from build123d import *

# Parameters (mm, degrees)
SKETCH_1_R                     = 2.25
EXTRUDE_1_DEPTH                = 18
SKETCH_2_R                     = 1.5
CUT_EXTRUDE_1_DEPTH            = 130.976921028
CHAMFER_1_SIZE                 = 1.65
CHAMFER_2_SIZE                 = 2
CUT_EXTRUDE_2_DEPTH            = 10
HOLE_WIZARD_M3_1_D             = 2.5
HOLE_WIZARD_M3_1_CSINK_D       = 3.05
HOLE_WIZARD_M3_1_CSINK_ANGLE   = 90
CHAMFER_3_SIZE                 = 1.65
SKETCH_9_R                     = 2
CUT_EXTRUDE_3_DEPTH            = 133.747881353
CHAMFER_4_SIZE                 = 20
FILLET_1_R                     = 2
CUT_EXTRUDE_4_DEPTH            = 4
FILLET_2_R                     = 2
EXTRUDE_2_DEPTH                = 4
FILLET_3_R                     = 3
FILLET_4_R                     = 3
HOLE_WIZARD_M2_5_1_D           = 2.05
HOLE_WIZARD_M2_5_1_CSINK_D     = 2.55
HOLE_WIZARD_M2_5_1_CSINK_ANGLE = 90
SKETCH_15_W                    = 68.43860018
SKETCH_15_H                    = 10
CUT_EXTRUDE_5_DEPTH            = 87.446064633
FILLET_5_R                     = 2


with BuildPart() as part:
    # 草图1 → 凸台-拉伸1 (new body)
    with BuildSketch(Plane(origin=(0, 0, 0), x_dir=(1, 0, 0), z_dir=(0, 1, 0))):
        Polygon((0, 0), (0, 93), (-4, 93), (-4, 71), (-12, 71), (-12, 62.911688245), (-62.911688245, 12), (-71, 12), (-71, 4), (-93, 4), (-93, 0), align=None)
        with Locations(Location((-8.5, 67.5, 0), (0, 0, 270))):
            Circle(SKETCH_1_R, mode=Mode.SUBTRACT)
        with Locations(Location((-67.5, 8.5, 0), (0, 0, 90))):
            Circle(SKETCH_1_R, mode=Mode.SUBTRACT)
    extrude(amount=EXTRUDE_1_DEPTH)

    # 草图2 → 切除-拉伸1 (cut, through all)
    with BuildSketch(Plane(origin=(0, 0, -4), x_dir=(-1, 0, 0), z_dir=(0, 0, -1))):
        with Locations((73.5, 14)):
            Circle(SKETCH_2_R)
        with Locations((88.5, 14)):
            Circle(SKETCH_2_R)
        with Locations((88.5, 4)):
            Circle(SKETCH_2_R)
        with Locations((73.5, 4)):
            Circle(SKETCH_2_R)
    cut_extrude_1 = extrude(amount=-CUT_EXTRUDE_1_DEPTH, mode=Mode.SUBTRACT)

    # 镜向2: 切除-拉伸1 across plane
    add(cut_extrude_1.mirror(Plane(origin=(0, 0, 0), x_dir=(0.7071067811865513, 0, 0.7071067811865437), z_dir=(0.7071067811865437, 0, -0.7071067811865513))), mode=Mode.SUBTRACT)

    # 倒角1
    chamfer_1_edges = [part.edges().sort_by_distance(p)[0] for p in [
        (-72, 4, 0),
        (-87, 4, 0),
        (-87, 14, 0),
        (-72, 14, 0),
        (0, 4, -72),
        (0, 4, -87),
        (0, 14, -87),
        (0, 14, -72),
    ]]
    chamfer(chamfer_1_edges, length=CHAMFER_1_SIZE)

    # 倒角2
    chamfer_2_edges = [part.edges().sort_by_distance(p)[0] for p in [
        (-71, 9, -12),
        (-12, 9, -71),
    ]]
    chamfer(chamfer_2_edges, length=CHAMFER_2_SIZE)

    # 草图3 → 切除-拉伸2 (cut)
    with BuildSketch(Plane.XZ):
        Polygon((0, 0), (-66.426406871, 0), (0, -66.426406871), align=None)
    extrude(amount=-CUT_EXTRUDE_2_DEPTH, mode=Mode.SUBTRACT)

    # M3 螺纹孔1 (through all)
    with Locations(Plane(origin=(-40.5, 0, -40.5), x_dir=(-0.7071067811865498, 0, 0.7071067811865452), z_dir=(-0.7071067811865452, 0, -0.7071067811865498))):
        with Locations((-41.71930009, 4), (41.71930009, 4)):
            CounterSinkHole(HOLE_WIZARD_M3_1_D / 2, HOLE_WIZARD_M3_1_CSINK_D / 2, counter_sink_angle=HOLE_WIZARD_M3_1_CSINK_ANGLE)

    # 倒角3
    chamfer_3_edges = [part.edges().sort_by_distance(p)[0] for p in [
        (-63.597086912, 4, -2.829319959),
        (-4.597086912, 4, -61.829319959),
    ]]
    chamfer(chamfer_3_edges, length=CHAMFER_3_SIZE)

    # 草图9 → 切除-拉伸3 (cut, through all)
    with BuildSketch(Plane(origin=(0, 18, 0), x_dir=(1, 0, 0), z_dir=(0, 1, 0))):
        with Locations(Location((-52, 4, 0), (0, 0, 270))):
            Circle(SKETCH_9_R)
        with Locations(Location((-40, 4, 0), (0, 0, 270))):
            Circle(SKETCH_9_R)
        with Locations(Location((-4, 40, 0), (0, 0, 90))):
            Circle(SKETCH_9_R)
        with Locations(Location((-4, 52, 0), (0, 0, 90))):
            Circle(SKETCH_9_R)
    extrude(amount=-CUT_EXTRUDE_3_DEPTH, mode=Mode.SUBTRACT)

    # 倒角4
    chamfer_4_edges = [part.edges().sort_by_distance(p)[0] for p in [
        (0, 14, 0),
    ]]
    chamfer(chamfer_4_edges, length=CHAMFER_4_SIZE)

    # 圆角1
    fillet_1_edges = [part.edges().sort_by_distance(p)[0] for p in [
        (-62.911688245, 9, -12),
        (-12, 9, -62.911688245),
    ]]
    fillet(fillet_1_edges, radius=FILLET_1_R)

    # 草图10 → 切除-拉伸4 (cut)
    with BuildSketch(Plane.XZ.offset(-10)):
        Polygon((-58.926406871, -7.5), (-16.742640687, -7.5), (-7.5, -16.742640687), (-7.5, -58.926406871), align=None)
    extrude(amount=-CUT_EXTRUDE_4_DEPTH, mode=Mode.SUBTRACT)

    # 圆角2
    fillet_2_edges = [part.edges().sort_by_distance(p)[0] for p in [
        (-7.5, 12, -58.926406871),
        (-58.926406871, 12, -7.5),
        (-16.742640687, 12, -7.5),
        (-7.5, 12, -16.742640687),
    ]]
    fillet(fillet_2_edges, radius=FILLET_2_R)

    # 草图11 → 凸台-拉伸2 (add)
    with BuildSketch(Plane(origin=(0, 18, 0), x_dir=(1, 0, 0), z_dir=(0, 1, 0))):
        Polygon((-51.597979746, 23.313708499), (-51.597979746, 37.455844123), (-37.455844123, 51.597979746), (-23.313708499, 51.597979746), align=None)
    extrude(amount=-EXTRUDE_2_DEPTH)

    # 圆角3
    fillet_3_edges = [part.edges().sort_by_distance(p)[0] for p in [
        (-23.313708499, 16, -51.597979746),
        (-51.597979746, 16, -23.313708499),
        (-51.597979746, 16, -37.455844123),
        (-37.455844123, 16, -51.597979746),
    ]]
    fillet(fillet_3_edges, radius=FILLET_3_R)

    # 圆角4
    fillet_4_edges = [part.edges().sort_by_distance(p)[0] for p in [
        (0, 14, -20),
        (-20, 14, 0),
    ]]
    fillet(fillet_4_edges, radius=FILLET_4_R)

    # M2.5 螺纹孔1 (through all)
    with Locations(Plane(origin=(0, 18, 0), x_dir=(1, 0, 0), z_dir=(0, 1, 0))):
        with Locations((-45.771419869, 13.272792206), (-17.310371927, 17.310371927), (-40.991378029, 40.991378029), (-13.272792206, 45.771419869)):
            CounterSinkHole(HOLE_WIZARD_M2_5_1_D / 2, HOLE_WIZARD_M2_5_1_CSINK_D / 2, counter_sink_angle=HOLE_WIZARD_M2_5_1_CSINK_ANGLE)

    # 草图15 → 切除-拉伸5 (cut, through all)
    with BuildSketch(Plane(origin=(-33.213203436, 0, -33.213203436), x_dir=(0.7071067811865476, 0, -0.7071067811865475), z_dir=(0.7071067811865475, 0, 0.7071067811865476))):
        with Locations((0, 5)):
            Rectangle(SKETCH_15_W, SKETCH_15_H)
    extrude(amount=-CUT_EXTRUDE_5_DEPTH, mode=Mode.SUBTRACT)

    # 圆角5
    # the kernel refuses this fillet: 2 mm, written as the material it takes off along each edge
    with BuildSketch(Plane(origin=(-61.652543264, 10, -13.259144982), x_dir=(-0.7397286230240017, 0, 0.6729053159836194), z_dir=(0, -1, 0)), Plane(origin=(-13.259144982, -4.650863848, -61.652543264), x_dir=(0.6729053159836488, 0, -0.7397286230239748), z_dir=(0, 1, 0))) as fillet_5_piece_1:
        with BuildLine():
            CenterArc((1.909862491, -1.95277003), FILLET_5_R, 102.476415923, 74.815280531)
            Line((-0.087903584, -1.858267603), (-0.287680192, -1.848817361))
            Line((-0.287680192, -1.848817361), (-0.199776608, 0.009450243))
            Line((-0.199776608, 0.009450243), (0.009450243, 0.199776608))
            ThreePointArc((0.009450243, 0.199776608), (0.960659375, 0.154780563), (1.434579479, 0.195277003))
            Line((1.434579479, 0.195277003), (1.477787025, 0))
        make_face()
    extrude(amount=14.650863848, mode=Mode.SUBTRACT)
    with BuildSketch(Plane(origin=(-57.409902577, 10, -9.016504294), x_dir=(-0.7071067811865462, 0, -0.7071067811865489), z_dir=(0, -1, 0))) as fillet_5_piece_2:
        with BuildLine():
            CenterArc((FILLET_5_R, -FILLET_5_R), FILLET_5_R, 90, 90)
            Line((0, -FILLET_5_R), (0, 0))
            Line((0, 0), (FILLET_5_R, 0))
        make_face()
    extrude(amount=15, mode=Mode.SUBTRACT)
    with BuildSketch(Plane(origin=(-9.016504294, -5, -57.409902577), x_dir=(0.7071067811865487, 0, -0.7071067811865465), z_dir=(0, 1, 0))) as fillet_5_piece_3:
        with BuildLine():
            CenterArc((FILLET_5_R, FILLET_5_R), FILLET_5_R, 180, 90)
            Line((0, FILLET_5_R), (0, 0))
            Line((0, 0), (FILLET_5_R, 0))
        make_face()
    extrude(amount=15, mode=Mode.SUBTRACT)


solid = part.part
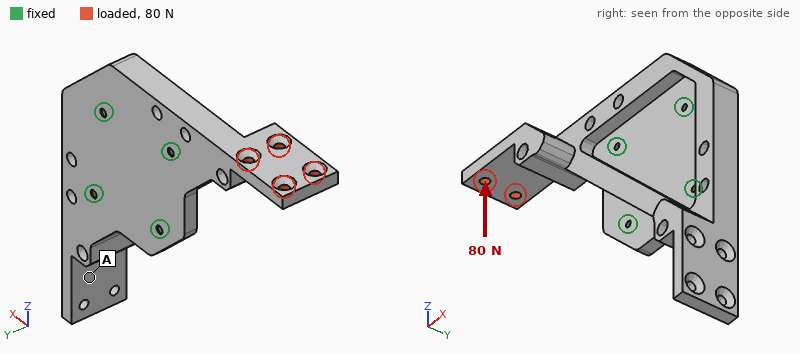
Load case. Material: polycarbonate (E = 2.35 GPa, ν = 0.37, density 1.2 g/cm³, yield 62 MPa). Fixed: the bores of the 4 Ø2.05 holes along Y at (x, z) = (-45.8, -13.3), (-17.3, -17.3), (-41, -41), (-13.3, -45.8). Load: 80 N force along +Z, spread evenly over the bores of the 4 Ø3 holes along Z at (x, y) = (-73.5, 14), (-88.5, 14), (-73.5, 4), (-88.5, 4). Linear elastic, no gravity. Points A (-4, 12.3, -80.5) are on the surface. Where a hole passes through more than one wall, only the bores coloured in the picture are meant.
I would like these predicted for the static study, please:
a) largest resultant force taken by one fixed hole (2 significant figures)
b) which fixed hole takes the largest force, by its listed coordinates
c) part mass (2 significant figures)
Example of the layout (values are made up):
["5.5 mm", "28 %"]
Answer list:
["80 N", "(-45.8, -13.3)", "26 g"]
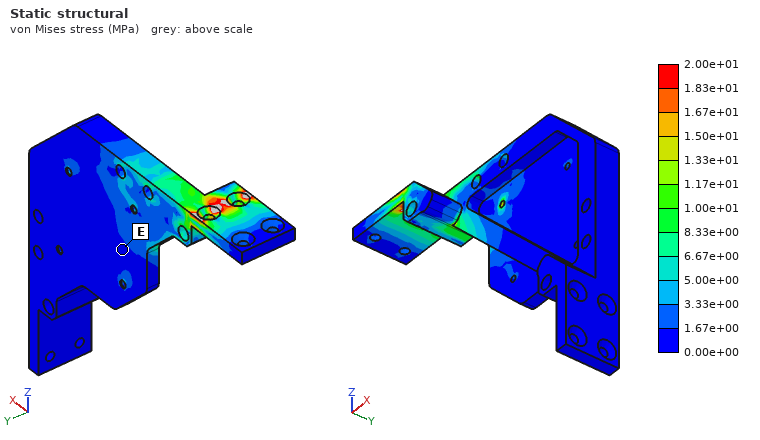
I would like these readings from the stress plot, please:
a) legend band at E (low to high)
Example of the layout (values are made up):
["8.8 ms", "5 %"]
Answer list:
["0.00e+00 to 1.67e+00 MPa"]
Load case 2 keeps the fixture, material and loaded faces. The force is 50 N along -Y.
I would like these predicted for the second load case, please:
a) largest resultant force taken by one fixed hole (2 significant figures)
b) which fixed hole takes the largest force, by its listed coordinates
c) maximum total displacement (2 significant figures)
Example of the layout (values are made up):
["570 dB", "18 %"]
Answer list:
["120 N", "(-45.8, -13.3)", "1.5 mm"]
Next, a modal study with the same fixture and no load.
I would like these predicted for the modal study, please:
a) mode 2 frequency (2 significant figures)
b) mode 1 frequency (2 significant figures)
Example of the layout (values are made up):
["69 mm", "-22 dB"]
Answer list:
["690 Hz", "690 Hz"]
